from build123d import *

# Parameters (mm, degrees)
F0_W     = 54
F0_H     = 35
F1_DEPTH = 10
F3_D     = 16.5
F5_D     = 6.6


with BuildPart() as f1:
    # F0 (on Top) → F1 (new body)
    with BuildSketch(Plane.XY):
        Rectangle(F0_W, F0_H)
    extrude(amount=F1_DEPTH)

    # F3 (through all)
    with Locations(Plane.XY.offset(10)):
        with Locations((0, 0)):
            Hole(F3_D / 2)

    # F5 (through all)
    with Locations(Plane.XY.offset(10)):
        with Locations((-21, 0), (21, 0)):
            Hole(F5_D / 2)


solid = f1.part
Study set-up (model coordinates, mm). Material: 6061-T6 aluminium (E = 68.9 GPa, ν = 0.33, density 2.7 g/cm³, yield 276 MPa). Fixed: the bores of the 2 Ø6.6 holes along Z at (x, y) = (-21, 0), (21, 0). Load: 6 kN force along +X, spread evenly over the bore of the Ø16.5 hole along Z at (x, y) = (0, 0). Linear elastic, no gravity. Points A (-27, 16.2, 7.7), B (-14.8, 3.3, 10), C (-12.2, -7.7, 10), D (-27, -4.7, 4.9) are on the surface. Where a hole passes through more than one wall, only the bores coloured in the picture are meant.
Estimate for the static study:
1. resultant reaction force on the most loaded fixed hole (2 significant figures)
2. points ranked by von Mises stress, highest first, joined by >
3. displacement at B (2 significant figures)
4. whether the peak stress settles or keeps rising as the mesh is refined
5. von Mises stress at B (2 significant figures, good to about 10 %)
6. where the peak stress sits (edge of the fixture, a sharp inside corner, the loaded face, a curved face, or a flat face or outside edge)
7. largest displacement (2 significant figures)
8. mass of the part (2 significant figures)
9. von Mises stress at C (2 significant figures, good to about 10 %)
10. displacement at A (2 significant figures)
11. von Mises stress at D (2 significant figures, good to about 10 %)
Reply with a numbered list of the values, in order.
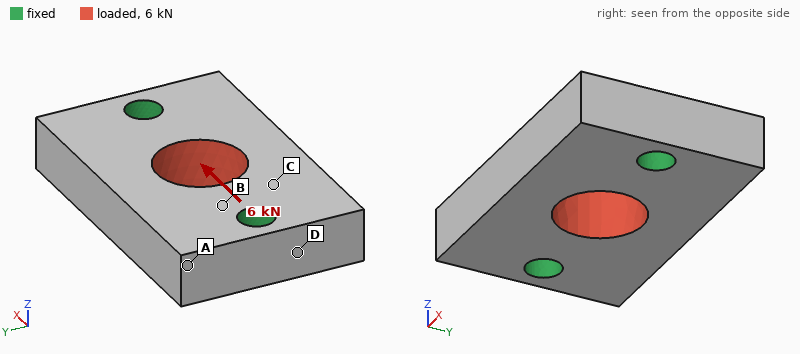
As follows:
1. 3.0 kN
2. B > C > D > A
3. 1.5 µm
4. keeps rising
5. 19 MPa
6. edge of the fixture
7. 5.0 µm
8. 43 g
9. 13 MPa
10. 3.4 µm
11. 7.5 MPa
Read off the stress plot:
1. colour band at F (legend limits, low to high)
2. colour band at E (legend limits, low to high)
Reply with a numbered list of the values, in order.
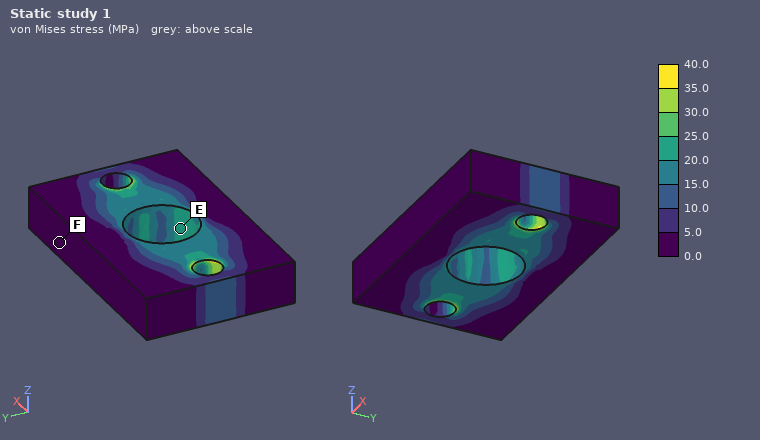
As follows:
1. 0.0 to 5.0 MPa
2. 20.0 to 25.0 MPa
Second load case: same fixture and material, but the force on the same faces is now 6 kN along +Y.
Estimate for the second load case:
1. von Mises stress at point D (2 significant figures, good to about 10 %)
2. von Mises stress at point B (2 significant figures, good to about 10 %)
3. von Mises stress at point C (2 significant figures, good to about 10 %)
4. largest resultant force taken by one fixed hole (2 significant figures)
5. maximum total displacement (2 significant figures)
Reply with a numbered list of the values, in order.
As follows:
1. 5.5 MPa
2. 24 MPa
3. 18 MPa
4. 3.0 kN
5. 9.7 µm
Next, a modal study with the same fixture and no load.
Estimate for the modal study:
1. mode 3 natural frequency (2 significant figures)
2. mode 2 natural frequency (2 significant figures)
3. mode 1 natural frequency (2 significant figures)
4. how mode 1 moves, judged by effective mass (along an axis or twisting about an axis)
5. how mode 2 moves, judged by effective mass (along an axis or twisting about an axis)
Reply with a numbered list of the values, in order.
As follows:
1. 26 kHz
2. 18 kHz
3. 16 kHz
4. twisting about X
5. along Z
